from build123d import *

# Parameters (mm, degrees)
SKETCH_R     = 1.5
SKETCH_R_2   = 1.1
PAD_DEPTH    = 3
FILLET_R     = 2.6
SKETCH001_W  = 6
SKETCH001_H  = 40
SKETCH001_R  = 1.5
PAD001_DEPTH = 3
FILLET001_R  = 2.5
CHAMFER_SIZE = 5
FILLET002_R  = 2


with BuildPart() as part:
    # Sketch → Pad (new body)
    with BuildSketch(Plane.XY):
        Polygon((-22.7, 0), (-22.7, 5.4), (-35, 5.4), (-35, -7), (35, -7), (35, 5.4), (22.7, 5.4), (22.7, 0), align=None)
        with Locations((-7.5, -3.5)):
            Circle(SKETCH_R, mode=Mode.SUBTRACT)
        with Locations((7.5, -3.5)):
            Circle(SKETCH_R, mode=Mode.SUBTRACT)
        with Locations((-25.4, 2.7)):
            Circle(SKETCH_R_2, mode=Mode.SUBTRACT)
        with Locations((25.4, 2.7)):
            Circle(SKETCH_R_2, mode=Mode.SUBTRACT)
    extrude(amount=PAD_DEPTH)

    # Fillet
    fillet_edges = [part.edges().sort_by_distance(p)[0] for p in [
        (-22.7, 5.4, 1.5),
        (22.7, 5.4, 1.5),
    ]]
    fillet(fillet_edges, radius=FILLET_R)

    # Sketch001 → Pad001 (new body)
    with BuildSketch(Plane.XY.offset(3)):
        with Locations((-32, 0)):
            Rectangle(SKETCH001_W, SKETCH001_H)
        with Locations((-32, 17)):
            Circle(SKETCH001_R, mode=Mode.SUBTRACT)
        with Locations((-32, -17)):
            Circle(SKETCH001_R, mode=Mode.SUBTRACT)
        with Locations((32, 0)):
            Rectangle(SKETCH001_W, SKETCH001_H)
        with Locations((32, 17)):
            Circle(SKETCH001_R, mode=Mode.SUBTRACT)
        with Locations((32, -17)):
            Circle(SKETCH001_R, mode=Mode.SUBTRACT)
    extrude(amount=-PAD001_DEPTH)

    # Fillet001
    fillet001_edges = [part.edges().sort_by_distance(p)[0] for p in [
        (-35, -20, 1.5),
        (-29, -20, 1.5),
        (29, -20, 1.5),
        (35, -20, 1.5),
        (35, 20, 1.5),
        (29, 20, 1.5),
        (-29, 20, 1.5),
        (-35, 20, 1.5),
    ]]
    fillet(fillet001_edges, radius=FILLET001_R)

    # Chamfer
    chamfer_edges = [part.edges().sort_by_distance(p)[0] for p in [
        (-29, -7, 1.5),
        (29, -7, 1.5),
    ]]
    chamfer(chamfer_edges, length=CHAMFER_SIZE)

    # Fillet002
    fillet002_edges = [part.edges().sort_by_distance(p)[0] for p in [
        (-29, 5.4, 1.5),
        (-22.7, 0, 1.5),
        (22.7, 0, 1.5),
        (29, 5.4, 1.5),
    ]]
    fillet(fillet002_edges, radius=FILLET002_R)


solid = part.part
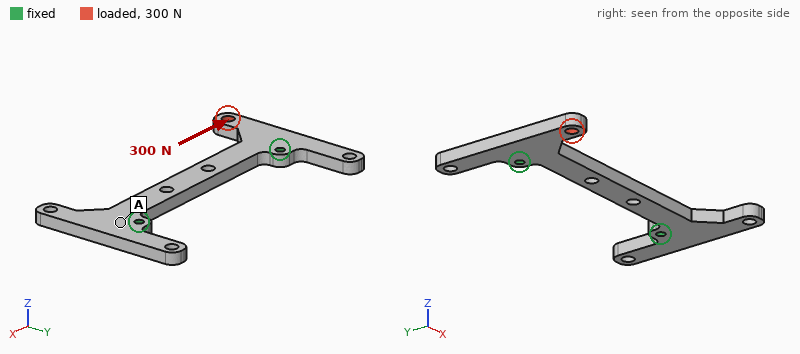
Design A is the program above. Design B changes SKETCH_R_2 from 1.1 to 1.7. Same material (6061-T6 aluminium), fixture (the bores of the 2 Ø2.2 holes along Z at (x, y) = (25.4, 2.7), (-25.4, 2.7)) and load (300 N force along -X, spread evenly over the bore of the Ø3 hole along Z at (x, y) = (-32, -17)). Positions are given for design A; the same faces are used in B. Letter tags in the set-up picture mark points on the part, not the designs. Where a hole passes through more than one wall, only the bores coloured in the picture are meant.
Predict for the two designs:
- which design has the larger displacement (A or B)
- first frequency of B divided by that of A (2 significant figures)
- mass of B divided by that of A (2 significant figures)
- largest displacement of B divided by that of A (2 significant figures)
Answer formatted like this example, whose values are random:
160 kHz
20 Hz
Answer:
A
1.1
0.99
0.82
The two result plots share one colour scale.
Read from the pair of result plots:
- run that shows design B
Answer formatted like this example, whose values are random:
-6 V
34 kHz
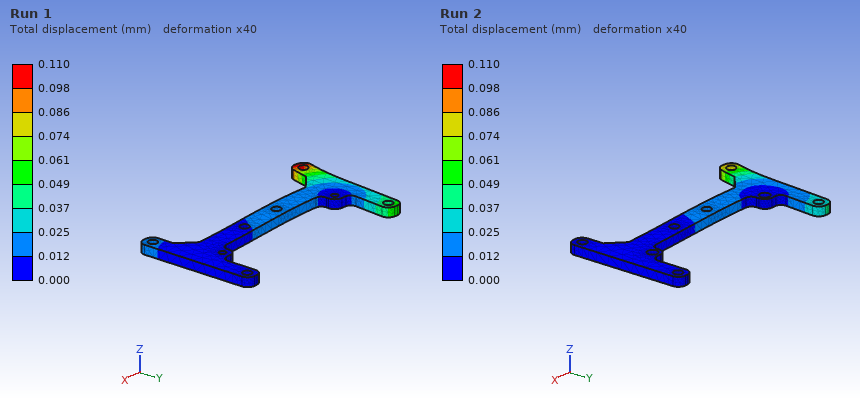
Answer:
Run 2
